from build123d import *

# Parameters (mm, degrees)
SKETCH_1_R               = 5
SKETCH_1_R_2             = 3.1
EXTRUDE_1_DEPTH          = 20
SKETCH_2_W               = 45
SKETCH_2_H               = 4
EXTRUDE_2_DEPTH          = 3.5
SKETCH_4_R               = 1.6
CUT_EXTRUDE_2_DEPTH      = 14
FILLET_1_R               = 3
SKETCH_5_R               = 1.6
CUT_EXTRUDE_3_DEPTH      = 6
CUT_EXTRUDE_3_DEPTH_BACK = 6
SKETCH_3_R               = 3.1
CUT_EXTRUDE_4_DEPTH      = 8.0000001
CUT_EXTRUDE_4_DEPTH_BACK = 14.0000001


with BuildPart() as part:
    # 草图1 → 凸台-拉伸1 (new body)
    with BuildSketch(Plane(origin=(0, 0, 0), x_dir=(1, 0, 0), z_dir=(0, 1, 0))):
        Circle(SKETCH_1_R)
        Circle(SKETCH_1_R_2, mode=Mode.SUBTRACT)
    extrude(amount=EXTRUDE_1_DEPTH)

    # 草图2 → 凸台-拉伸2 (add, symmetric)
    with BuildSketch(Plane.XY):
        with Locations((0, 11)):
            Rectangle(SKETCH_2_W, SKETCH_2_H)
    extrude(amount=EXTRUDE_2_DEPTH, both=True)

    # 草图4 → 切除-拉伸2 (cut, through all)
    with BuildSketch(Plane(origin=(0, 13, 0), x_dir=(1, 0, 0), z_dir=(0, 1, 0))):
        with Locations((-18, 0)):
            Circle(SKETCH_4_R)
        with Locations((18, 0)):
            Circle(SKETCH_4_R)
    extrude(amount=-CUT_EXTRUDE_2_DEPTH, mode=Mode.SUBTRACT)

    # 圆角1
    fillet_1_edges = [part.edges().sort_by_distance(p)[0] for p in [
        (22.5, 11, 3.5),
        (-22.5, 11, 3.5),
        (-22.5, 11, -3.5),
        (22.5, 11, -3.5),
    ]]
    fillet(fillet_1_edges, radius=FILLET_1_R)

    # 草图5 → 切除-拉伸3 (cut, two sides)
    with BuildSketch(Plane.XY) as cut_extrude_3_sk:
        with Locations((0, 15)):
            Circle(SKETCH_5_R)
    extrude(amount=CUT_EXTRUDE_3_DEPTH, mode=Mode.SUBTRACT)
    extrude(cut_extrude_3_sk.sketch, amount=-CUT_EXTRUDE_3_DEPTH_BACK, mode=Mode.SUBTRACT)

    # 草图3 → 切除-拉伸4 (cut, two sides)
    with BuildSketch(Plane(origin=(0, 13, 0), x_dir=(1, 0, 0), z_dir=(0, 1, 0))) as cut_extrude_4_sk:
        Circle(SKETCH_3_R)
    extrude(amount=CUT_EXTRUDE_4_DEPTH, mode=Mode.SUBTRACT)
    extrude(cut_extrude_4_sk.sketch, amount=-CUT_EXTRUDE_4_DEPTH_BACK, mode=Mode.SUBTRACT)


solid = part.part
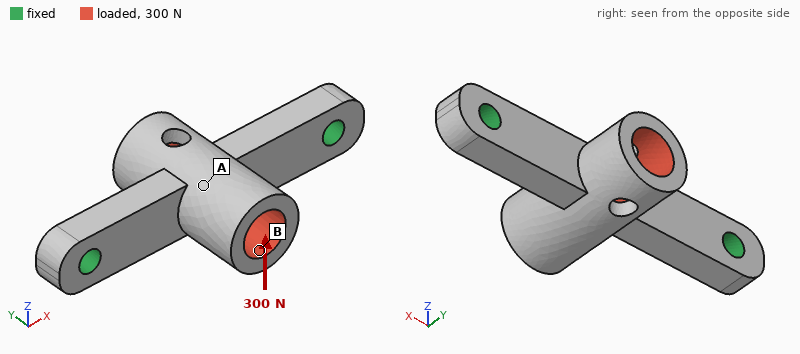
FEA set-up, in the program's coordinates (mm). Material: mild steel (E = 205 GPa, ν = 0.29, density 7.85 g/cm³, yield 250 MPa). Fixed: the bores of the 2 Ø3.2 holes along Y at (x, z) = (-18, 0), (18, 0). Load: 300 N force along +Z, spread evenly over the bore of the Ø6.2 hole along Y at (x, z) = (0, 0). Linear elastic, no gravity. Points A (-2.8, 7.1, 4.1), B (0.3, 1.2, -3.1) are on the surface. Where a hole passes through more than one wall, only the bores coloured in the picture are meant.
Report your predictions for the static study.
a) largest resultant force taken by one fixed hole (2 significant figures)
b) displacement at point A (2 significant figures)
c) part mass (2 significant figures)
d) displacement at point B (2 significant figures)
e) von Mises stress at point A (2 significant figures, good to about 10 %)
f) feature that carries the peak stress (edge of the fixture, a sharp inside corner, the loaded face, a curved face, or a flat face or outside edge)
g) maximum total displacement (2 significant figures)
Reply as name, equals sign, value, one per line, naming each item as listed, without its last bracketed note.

largest resultant force taken by one fixed hole = 150 N
displacement at point A = 5.2 µm
part mass = 14 g
displacement at point B = 7.4 µm
von Mises stress at point A = 7.7 MPa
feature that carries the peak stress = edge of the fixture
maximum total displacement = 8.0 µm
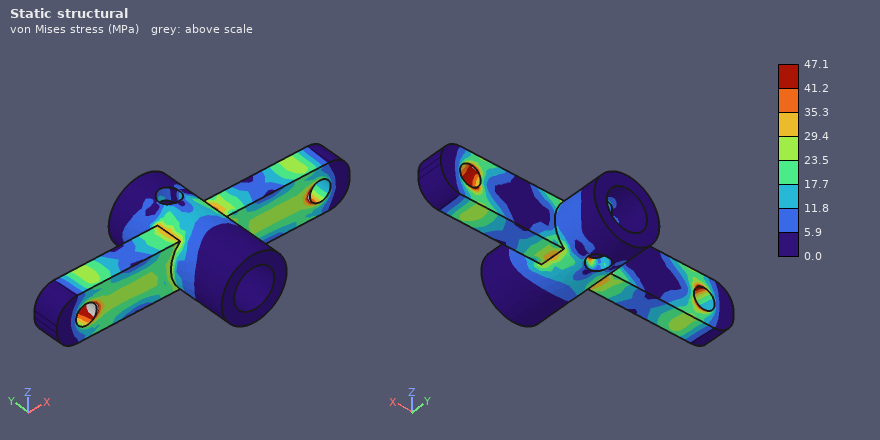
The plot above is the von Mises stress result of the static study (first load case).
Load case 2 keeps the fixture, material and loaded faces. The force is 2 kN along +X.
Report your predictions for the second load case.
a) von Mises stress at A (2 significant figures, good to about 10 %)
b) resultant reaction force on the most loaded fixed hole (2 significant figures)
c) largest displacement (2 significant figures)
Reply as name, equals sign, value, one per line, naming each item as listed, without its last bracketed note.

von Mises stress at A = 28 MPa
resultant reaction force on the most loaded fixed hole = 1.0 kN
largest displacement = 11 µm
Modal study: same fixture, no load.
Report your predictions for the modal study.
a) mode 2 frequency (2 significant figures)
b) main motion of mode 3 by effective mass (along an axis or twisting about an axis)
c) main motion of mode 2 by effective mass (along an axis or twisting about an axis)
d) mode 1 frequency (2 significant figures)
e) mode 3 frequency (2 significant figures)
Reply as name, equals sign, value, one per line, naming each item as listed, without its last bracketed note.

mode 2 frequency = 12 kHz
main motion of mode 3 by effective mass = along Z
main motion of mode 2 by effective mass = along Y
mode 1 frequency = 9400 Hz
mode 3 frequency = 15 kHz
